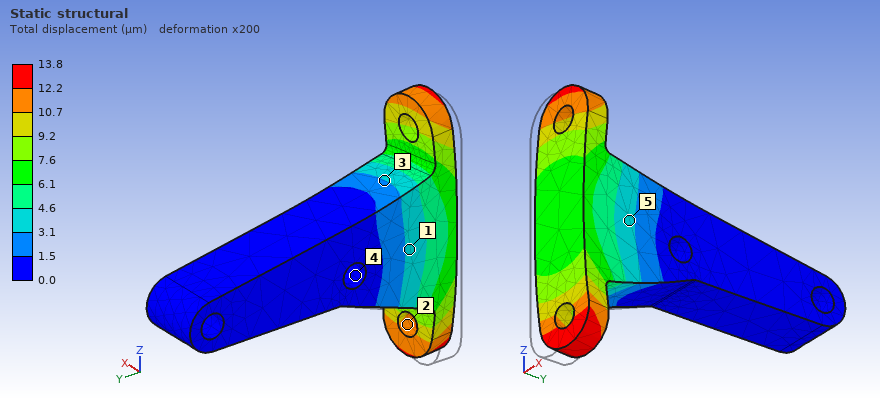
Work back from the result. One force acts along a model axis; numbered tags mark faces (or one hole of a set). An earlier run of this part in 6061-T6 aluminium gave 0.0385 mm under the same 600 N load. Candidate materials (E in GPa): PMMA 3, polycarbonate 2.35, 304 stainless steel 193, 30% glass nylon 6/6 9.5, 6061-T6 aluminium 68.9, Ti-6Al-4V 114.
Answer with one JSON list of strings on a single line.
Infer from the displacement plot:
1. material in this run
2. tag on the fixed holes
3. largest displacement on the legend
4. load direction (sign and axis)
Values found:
["304 stainless steel", "4", "13.8 µm", "+X"]
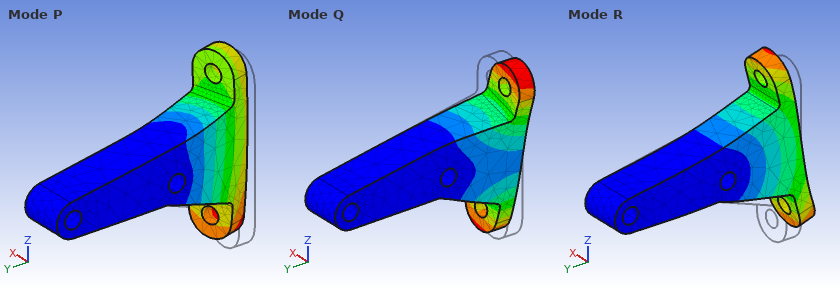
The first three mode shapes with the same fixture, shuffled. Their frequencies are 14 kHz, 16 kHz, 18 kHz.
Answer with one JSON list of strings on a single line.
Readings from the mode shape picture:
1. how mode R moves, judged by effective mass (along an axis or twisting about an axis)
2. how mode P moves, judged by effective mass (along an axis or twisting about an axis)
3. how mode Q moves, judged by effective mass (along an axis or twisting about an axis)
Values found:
["along Z", "along X", "twisting about Y"]
